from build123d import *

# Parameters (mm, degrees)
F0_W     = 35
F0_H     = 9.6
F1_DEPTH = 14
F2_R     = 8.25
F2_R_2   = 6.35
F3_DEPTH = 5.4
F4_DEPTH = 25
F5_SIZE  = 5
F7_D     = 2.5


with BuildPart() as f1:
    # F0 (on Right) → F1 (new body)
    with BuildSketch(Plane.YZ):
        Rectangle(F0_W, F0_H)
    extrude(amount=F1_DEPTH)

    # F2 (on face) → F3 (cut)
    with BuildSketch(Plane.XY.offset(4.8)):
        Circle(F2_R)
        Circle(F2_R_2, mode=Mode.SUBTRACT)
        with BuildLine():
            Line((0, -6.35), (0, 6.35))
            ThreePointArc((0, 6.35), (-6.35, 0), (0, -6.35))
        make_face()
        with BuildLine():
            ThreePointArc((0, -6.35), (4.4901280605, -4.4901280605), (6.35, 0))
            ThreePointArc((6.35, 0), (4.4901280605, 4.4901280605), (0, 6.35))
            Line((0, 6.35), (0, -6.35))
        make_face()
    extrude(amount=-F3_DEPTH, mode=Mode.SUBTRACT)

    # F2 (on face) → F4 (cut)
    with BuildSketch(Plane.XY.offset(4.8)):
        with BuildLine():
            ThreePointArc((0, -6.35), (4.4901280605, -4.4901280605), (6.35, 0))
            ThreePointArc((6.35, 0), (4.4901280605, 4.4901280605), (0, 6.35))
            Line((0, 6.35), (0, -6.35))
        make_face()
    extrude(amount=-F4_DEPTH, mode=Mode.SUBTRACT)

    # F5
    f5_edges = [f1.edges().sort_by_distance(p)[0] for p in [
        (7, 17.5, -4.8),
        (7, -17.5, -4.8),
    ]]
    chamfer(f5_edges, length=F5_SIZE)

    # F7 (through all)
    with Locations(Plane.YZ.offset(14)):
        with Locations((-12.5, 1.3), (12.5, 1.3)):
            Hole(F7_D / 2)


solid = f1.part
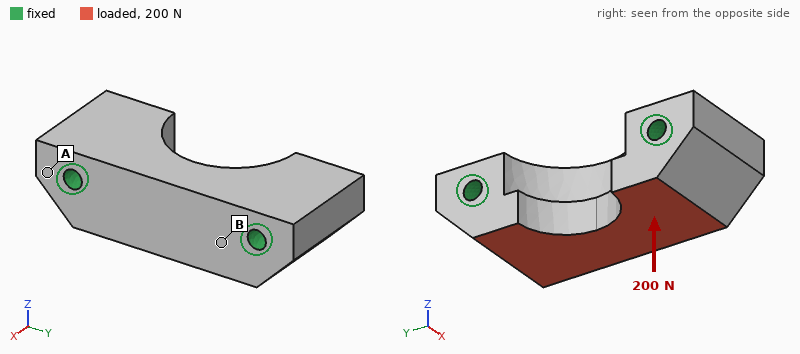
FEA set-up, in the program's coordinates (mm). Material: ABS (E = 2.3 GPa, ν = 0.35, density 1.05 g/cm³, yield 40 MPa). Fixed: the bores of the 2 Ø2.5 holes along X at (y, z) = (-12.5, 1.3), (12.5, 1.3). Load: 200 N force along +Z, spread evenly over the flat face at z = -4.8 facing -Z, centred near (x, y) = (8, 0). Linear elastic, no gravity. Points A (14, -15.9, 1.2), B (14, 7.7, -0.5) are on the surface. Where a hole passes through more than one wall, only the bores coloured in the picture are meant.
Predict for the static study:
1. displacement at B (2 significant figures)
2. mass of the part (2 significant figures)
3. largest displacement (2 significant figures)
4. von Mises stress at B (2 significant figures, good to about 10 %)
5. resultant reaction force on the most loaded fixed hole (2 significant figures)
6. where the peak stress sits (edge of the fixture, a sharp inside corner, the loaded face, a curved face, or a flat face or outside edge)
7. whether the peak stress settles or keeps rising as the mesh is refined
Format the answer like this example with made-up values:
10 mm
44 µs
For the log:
9.5 µm
3.5 g
19 µm
1.8 MPa
110 N
edge of the fixture
keeps rising
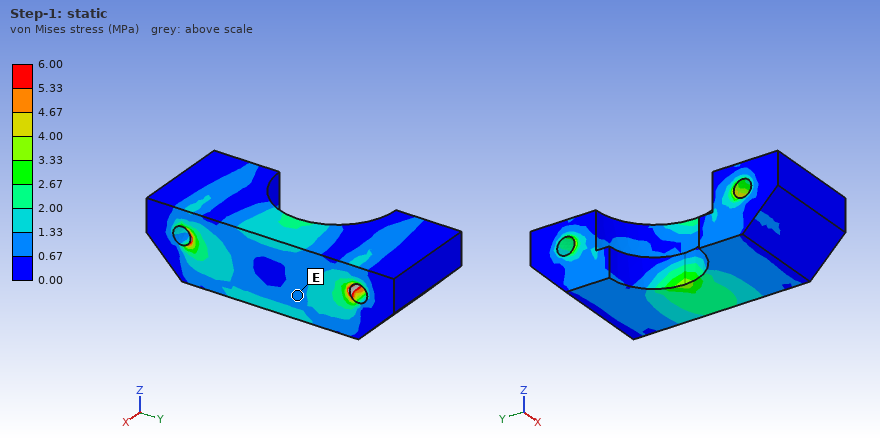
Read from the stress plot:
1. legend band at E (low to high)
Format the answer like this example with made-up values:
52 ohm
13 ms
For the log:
0.67 to 1.33 MPa
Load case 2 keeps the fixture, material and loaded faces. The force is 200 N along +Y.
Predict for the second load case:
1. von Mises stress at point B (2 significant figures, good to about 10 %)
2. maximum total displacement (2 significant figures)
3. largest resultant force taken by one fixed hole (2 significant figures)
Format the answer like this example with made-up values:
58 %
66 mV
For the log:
1.1 MPa
13 µm
110 N
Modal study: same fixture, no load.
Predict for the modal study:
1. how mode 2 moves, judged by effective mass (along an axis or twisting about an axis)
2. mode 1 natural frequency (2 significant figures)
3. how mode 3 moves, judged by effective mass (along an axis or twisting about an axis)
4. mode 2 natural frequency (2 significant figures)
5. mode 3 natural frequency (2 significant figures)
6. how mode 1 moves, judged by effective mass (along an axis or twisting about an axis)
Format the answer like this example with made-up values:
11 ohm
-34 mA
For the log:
along X
12 kHz
twisting about Y
16 kHz
21 kHz
along Z
